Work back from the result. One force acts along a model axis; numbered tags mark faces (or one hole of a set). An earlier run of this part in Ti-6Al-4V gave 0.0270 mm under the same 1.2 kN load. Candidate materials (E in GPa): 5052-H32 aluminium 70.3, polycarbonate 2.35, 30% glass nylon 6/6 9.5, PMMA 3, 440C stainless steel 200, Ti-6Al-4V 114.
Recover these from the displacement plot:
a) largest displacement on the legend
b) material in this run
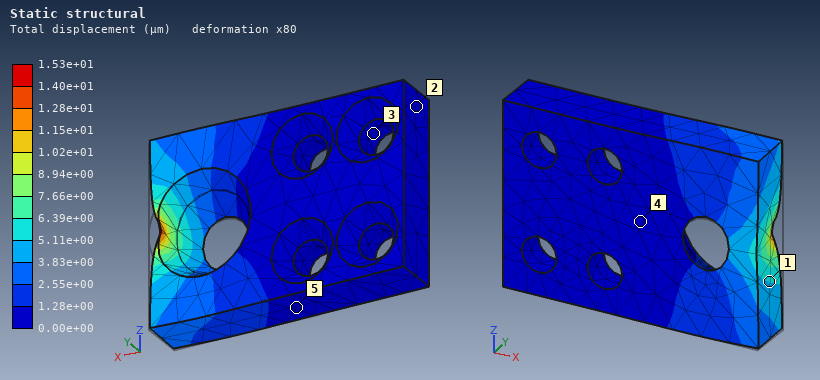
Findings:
1.53e+01 µm
440C stainless steel
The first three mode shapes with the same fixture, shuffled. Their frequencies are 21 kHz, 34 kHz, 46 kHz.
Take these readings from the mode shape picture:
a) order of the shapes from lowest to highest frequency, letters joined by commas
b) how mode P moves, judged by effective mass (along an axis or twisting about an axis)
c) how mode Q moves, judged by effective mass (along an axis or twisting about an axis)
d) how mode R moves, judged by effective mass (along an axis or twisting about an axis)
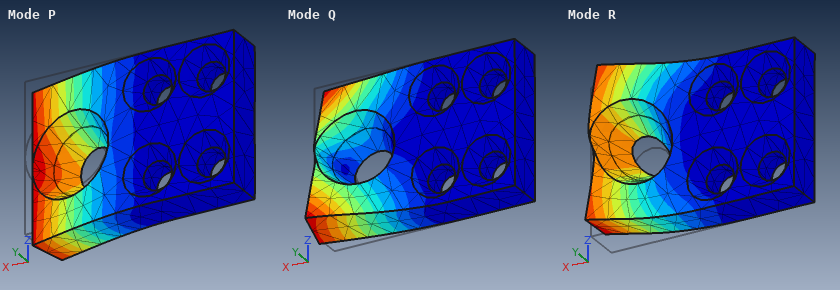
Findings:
P, Q, R
along Y
twisting about X
along Z
